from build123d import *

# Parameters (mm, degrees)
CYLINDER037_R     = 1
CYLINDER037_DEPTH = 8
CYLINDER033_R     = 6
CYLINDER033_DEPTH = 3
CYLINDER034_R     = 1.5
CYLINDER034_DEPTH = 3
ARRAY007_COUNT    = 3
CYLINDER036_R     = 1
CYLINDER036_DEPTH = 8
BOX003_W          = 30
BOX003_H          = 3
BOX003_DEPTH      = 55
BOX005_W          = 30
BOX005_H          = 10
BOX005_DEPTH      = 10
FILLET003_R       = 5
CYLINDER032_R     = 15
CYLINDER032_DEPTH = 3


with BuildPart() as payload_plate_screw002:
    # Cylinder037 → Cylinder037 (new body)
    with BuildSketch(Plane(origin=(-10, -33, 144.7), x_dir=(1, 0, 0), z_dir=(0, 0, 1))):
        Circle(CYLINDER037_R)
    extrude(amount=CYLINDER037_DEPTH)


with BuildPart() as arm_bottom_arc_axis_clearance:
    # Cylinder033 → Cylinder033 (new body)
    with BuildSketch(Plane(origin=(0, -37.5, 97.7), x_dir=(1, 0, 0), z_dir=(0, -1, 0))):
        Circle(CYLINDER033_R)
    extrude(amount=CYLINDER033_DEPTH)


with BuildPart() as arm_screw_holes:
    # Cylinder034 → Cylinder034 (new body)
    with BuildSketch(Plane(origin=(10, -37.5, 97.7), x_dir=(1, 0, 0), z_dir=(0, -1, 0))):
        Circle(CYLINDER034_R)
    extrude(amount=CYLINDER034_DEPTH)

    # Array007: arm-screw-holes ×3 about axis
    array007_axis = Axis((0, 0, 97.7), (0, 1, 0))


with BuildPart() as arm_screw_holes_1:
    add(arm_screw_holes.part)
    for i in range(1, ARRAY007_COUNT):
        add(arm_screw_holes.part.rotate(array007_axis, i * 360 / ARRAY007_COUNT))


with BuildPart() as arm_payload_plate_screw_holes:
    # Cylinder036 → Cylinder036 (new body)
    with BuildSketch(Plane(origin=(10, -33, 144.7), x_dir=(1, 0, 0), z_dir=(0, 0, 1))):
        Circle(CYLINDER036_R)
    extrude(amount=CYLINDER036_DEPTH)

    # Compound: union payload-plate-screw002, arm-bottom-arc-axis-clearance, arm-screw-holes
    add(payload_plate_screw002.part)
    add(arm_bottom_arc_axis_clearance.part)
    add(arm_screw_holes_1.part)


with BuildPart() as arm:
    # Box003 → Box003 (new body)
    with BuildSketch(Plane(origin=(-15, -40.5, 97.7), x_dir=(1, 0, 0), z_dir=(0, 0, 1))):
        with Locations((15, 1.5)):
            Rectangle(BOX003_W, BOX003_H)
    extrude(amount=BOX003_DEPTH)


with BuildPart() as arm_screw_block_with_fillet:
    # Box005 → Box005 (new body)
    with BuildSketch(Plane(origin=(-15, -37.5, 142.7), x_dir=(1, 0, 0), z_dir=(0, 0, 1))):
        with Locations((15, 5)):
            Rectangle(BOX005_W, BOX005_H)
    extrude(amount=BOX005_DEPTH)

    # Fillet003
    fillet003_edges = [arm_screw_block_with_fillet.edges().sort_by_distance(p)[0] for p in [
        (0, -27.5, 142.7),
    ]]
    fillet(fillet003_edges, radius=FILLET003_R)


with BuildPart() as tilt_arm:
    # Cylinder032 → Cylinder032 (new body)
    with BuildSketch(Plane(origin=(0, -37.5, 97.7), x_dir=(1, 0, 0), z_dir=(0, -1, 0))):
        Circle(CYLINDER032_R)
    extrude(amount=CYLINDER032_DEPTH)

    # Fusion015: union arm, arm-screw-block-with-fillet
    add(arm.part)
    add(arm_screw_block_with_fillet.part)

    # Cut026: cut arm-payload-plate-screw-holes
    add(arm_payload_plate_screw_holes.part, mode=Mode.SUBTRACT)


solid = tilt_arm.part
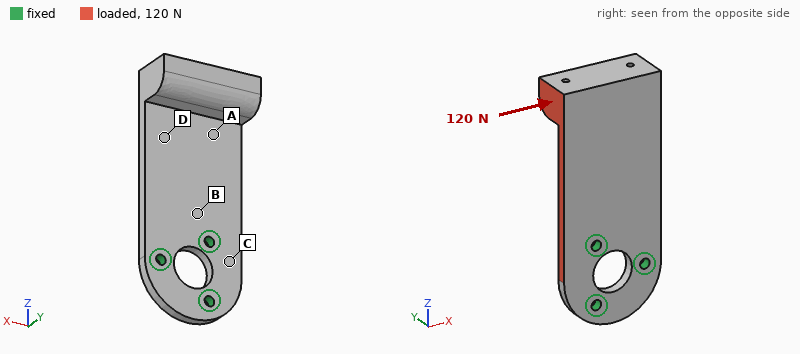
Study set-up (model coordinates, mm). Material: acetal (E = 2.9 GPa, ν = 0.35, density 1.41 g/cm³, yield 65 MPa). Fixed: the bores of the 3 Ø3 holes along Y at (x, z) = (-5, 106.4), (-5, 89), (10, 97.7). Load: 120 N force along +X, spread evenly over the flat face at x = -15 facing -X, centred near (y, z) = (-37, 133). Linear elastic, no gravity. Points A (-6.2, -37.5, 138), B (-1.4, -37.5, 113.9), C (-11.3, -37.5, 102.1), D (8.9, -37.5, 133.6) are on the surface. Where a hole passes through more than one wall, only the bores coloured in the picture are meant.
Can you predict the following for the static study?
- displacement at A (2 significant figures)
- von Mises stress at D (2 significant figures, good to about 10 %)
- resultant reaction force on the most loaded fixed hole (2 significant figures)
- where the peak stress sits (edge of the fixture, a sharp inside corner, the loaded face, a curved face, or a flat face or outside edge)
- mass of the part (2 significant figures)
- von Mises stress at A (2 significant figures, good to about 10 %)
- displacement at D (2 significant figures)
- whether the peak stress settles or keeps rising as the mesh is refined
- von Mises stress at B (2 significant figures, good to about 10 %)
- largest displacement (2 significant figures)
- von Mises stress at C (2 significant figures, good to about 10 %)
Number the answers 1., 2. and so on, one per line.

1. 0.21 mm
2. 6.1 MPa
3. 190 N
4. edge of the fixture
5. 12 g
6. 5.2 MPa
7. 0.35 mm
8. keeps rising
9. 8.0 MPa
10. 0.83 mm
11. 2.5 MPa
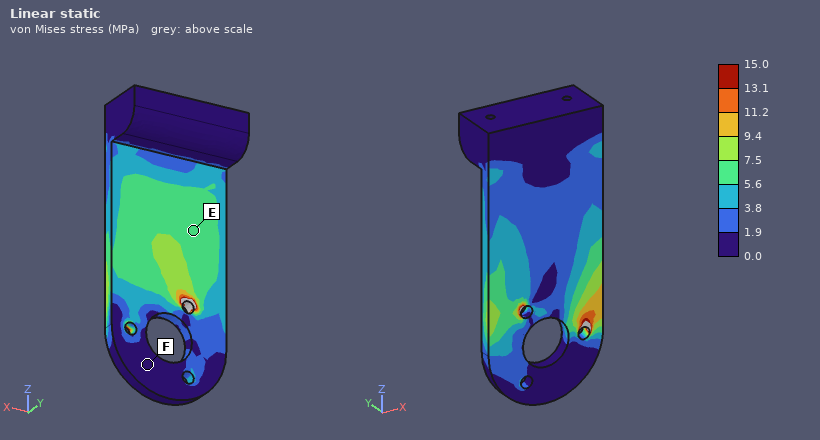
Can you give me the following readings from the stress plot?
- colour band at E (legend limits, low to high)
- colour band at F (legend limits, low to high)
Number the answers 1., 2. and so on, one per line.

1. 5.6 to 7.5 MPa
2. 0.0 to 1.9 MPa
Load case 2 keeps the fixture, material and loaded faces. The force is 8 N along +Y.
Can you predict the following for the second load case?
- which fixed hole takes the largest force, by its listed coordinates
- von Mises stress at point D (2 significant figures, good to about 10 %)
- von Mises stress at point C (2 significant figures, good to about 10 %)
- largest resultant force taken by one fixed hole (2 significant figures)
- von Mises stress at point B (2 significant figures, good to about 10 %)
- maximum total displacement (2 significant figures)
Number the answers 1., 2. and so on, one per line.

1. (-5, 106.4)
2. 1.8 MPa
3. 1.3 MPa
4. 15 N
5. 3.9 MPa
6. 0.84 mm
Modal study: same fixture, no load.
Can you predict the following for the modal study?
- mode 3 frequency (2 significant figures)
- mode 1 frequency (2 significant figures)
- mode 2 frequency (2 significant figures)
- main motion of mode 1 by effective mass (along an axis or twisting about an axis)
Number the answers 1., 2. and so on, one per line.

1. 1200 Hz
2. 170 Hz
3. 560 Hz
4. along Y
